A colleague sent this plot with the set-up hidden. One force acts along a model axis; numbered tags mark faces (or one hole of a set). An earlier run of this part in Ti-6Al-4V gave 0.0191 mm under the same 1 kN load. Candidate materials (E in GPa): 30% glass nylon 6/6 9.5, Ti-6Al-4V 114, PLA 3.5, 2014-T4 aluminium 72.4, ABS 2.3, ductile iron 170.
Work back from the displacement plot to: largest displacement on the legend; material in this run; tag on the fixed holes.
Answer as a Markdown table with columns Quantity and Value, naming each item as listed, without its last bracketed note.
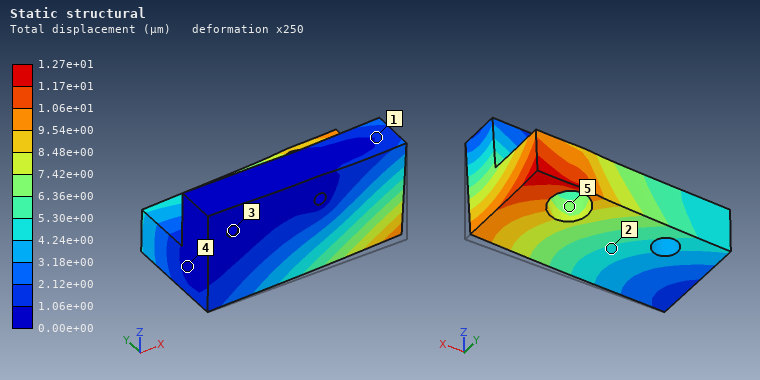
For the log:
| Quantity | Value |
|---|---|
| largest displacement on the legend | 1.27e+01 µm |
| material in this run | ductile iron |
| tag on the fixed holes | 3 |
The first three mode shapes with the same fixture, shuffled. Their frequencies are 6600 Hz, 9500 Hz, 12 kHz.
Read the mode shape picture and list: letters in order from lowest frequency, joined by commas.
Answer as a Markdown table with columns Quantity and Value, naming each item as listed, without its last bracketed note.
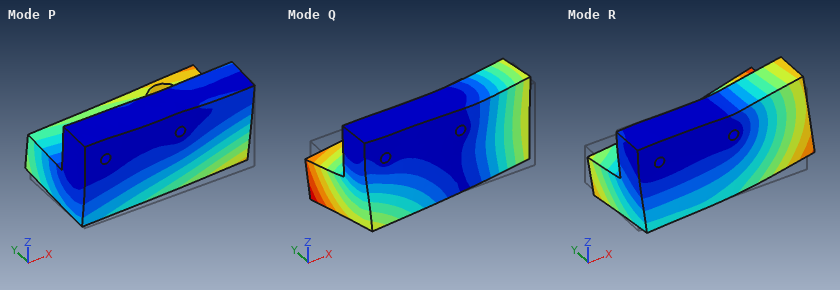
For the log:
| Quantity | Value |
|---|---|
| letters in order from lowest frequency, joined by commas | P, Q, R |
